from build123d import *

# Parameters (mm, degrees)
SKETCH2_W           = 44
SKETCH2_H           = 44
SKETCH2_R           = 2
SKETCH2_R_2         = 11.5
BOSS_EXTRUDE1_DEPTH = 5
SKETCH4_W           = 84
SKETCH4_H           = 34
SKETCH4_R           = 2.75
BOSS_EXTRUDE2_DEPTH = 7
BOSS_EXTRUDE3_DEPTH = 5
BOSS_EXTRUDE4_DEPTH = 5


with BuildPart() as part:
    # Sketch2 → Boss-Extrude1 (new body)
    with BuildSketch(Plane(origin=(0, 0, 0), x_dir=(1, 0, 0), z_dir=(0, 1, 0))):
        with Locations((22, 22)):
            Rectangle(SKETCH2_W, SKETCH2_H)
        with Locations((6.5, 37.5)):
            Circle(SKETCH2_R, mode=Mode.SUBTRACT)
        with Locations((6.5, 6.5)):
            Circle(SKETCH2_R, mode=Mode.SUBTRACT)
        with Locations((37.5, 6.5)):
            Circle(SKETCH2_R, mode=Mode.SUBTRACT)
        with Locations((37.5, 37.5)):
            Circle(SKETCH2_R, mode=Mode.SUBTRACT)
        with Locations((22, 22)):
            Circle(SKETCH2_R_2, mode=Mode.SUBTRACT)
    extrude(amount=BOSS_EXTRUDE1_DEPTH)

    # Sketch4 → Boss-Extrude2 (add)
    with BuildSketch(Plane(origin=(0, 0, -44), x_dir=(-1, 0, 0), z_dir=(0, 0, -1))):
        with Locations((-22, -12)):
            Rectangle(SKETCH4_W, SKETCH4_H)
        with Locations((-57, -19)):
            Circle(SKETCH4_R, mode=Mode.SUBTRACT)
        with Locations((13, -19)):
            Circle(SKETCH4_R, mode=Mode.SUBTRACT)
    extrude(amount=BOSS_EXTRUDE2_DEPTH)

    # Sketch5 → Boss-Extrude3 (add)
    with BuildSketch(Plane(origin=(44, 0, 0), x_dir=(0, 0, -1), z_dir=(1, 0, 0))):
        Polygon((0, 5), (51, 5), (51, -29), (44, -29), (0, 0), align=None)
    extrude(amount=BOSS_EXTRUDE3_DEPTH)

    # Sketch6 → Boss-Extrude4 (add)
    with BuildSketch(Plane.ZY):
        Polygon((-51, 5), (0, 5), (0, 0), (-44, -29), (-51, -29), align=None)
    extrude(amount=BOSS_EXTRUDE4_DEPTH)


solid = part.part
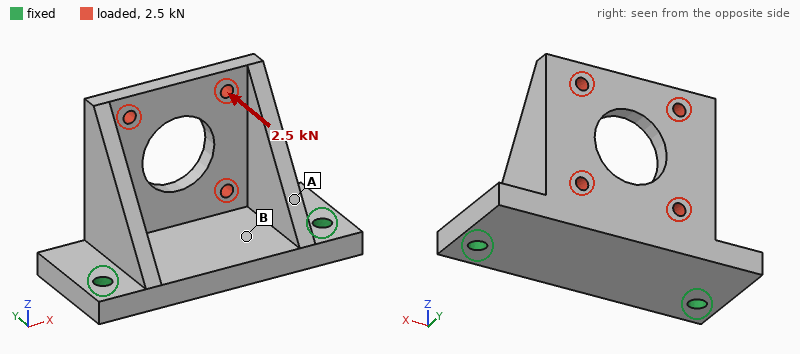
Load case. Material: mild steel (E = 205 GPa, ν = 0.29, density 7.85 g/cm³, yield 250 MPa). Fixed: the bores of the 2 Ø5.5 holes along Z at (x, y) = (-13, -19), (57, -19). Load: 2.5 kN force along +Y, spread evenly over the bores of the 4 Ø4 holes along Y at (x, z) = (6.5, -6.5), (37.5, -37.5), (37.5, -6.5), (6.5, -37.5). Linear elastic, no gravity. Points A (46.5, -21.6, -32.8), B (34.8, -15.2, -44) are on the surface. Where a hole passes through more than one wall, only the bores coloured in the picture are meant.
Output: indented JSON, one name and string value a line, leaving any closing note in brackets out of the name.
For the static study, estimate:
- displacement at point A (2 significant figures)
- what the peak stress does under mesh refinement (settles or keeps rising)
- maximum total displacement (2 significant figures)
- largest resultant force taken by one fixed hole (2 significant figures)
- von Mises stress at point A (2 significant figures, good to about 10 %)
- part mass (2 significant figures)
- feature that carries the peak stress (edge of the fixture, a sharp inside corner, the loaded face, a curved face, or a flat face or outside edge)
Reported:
{
  "displacement at point A": "0.025 mm",
  "what the peak stress does under mesh refinement": "keeps rising",
  "maximum total displacement": "0.12 mm",
  "largest resultant force taken by one fixed hole": "1.3 kN",
  "von Mises stress at point A": "53 MPa",
  "part mass": "280 g",
  "feature that carries the peak stress": "edge of the fixture"
}
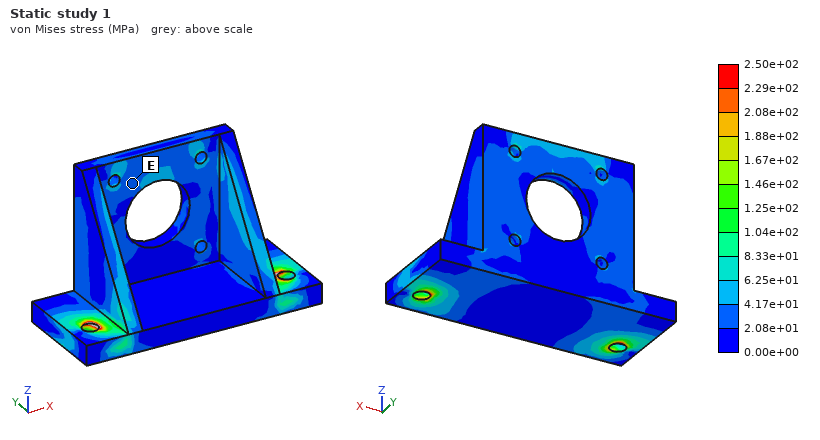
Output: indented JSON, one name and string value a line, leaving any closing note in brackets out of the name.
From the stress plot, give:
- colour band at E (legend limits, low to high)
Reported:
{
  "colour band at E": "2.08e+01 to 4.17e+01 MPa"
}
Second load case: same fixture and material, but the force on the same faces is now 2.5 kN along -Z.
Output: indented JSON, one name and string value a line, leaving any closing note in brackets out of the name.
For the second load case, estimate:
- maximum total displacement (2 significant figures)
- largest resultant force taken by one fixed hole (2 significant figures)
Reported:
{
  "maximum total displacement": "72 µm",
  "largest resultant force taken by one fixed hole": "1.3 kN"
}
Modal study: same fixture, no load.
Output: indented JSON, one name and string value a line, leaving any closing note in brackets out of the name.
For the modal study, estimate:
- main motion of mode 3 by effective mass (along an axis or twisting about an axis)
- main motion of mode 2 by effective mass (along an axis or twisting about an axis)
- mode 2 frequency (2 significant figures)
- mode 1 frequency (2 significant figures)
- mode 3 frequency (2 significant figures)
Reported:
{
  "main motion of mode 3 by effective mass": "along Z",
  "main motion of mode 2 by effective mass": "along X",
  "mode 2 frequency": "4200 Hz",
  "mode 1 frequency": "2600 Hz",
  "mode 3 frequency": "7300 Hz"
}
